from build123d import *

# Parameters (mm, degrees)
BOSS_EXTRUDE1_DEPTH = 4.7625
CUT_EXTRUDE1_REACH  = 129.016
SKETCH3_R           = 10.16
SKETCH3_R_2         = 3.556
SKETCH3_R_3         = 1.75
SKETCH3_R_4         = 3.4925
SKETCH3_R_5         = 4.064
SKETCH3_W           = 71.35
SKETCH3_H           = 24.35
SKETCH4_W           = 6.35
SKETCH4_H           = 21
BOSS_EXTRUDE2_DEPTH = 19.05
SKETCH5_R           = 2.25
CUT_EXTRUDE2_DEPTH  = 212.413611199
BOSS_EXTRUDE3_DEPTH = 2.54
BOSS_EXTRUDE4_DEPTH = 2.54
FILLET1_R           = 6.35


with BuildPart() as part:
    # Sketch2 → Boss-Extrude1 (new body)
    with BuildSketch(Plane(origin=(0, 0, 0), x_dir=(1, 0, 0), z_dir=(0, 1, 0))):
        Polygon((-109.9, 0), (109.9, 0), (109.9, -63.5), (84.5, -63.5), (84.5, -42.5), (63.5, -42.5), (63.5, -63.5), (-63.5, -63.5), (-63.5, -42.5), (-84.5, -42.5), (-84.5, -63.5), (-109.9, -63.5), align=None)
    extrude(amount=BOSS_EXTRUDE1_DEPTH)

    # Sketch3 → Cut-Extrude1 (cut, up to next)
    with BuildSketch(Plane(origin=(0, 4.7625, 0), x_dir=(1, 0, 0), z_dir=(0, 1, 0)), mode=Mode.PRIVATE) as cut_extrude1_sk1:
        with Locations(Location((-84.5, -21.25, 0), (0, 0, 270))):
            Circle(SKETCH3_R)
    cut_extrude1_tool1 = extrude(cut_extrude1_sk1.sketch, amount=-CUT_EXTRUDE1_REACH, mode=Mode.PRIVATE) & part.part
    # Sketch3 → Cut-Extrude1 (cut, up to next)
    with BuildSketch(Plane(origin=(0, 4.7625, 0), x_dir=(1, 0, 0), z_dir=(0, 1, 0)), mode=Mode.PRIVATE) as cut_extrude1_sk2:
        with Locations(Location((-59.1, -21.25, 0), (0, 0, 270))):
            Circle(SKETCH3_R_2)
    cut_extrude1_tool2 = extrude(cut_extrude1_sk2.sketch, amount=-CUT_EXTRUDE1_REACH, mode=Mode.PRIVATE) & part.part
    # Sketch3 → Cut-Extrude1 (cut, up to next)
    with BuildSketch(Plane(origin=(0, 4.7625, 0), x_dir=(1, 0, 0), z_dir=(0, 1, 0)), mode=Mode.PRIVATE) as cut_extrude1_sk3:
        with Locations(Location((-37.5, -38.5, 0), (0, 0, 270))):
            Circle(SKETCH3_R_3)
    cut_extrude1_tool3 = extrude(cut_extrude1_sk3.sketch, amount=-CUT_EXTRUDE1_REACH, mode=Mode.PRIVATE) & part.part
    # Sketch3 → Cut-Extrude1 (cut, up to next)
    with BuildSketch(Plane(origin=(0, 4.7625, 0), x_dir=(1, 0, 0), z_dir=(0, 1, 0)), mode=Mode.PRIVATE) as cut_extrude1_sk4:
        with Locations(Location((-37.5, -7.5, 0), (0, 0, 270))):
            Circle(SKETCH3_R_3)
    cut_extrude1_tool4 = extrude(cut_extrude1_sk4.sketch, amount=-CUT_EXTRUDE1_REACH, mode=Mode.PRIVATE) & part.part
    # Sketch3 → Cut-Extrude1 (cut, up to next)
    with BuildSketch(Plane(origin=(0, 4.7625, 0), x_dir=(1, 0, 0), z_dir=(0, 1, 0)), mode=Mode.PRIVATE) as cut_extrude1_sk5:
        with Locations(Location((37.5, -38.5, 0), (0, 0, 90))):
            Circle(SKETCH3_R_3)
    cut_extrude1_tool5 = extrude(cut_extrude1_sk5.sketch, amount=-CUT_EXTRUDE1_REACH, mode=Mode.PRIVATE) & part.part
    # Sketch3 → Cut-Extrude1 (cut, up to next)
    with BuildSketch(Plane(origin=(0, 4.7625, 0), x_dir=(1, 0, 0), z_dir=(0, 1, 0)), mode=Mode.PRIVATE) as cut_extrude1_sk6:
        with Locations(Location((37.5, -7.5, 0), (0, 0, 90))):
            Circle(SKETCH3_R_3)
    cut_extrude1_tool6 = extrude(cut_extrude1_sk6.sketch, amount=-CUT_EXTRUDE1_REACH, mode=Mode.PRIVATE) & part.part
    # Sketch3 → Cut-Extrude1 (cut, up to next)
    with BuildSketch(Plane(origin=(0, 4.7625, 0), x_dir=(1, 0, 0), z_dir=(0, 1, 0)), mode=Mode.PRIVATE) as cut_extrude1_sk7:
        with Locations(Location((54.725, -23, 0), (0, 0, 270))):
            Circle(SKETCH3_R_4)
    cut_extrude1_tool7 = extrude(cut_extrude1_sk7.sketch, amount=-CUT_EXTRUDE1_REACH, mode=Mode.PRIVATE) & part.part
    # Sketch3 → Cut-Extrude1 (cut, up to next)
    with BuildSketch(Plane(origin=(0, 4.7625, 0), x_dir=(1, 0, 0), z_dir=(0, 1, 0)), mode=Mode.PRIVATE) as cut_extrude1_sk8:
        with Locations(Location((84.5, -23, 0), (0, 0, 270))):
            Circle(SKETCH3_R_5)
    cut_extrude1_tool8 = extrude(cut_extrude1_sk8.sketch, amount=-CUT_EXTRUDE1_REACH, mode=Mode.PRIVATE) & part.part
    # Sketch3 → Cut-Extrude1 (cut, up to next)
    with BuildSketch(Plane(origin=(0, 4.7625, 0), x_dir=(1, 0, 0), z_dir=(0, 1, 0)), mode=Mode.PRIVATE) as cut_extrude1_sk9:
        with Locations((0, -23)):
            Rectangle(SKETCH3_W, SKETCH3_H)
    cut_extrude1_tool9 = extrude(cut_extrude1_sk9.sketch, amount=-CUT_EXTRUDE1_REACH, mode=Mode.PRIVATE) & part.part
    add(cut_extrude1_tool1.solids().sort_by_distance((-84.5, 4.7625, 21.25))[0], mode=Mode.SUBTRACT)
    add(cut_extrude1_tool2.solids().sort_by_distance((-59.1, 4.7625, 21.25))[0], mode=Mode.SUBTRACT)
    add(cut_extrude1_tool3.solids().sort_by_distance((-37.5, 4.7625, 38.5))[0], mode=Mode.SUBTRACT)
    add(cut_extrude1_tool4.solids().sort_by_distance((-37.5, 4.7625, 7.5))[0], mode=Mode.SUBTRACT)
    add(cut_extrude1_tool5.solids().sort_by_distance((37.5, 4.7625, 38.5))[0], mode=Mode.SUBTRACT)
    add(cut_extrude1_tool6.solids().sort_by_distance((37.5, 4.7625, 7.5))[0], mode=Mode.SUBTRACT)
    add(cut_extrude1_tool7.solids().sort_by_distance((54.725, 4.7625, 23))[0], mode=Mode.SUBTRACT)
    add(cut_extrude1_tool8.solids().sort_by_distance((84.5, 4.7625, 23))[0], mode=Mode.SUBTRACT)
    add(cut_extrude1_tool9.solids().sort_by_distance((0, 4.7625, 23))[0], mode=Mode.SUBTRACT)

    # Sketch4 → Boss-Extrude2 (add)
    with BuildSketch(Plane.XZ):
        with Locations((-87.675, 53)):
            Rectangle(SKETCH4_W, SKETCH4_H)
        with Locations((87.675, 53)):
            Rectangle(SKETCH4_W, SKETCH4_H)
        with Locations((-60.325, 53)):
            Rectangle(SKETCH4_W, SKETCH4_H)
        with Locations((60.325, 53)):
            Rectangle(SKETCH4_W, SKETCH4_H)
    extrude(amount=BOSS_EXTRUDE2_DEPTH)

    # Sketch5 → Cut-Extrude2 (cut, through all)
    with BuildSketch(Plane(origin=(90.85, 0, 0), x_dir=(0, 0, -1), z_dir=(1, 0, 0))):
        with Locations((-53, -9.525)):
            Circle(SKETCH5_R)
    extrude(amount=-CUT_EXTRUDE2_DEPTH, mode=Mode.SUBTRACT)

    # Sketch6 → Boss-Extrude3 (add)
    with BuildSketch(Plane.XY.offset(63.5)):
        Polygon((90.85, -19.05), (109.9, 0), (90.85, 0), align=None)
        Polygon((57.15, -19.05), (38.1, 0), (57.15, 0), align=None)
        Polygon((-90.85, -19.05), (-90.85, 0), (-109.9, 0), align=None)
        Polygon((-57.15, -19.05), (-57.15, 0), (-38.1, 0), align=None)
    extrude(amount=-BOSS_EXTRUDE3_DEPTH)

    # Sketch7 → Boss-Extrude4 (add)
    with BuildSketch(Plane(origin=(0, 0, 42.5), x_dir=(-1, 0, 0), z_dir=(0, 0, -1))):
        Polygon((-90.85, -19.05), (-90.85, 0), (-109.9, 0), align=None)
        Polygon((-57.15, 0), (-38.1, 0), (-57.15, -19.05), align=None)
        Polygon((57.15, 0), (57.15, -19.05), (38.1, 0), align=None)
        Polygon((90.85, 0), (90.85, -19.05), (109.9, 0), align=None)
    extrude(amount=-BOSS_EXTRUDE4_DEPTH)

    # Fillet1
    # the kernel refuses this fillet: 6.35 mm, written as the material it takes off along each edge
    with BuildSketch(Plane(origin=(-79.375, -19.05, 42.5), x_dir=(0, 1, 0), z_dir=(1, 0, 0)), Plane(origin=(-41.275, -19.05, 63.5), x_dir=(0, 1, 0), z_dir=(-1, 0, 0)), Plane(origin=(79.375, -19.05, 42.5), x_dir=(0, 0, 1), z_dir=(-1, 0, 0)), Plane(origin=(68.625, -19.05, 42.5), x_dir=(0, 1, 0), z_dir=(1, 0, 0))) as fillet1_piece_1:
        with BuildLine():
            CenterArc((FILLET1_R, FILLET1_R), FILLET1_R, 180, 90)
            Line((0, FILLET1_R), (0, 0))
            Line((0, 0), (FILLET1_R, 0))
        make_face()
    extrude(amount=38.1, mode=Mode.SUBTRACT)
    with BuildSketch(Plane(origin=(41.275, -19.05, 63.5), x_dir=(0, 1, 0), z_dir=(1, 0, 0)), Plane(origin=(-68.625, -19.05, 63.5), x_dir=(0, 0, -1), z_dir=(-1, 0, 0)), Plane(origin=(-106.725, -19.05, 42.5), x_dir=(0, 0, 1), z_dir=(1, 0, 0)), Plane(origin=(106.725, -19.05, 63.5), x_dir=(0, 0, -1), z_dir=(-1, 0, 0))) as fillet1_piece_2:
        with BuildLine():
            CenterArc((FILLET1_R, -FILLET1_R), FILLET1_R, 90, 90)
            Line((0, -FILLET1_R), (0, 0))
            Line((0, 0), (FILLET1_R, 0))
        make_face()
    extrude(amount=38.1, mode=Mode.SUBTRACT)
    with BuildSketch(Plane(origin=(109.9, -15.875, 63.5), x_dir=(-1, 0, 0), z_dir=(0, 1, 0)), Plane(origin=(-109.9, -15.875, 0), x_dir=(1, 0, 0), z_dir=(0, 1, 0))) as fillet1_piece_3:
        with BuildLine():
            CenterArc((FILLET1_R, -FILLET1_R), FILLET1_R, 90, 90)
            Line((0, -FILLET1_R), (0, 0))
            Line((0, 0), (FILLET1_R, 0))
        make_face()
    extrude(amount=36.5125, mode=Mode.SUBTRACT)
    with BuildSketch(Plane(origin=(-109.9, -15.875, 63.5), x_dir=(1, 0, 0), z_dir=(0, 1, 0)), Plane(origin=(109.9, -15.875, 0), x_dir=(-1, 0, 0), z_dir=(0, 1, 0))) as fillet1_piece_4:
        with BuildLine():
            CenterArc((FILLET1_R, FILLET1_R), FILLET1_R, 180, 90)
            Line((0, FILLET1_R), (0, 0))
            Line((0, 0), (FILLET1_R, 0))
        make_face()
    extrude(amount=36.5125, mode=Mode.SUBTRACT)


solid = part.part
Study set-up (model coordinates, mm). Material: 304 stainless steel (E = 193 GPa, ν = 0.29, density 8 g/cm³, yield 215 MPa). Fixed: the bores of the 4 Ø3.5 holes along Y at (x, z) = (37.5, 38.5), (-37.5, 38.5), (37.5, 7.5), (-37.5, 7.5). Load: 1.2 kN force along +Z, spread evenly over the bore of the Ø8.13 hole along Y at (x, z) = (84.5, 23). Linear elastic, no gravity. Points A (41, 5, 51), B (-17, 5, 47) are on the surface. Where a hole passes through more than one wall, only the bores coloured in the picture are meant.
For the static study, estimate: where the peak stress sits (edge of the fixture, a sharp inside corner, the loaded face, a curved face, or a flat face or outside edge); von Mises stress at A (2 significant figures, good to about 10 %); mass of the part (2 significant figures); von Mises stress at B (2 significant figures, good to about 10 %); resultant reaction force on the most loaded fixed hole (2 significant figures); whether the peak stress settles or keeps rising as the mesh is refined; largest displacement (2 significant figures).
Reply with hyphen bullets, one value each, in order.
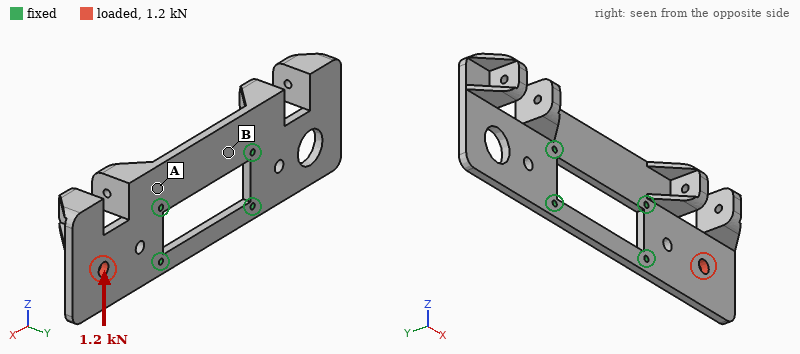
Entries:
- edge of the fixture
- 9.2 MPa
- 510 g
- 3.4 MPa
- 1.4 kN
- keeps rising
- 16 µm
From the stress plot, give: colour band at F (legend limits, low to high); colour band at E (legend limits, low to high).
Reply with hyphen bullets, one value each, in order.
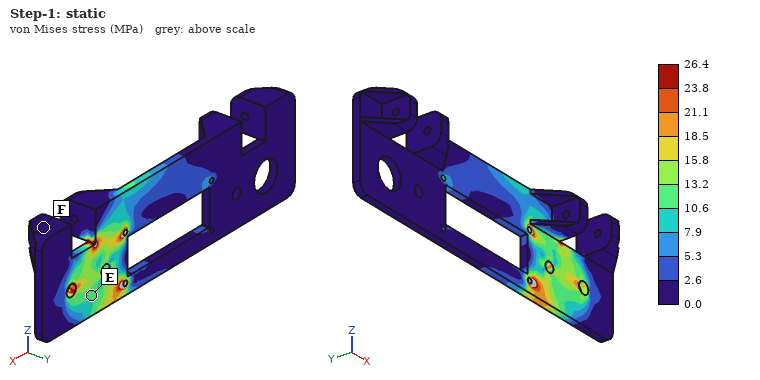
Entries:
- 0.0 to 2.6 MPa
- 10.6 to 13.2 MPa
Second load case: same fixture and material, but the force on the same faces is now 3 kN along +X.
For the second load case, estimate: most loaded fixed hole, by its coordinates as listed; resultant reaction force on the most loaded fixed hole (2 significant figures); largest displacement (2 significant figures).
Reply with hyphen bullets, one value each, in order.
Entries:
- (37.5, 7.5)
- 1.6 kN
- 5.9 µm
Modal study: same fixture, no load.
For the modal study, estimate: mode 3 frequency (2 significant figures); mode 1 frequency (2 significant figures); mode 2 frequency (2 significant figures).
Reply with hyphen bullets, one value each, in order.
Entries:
- 1200 Hz
- 560 Hz
- 570 Hz
